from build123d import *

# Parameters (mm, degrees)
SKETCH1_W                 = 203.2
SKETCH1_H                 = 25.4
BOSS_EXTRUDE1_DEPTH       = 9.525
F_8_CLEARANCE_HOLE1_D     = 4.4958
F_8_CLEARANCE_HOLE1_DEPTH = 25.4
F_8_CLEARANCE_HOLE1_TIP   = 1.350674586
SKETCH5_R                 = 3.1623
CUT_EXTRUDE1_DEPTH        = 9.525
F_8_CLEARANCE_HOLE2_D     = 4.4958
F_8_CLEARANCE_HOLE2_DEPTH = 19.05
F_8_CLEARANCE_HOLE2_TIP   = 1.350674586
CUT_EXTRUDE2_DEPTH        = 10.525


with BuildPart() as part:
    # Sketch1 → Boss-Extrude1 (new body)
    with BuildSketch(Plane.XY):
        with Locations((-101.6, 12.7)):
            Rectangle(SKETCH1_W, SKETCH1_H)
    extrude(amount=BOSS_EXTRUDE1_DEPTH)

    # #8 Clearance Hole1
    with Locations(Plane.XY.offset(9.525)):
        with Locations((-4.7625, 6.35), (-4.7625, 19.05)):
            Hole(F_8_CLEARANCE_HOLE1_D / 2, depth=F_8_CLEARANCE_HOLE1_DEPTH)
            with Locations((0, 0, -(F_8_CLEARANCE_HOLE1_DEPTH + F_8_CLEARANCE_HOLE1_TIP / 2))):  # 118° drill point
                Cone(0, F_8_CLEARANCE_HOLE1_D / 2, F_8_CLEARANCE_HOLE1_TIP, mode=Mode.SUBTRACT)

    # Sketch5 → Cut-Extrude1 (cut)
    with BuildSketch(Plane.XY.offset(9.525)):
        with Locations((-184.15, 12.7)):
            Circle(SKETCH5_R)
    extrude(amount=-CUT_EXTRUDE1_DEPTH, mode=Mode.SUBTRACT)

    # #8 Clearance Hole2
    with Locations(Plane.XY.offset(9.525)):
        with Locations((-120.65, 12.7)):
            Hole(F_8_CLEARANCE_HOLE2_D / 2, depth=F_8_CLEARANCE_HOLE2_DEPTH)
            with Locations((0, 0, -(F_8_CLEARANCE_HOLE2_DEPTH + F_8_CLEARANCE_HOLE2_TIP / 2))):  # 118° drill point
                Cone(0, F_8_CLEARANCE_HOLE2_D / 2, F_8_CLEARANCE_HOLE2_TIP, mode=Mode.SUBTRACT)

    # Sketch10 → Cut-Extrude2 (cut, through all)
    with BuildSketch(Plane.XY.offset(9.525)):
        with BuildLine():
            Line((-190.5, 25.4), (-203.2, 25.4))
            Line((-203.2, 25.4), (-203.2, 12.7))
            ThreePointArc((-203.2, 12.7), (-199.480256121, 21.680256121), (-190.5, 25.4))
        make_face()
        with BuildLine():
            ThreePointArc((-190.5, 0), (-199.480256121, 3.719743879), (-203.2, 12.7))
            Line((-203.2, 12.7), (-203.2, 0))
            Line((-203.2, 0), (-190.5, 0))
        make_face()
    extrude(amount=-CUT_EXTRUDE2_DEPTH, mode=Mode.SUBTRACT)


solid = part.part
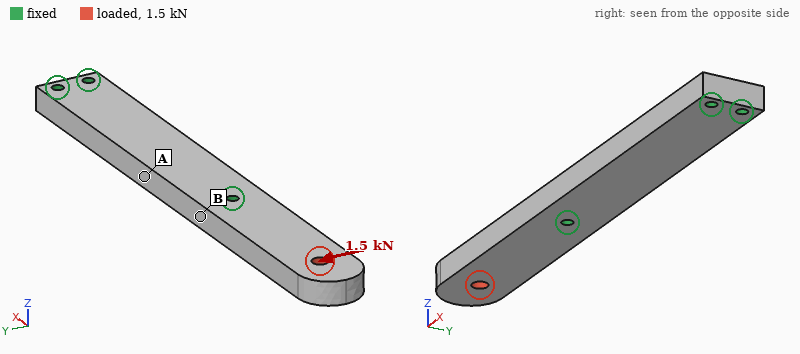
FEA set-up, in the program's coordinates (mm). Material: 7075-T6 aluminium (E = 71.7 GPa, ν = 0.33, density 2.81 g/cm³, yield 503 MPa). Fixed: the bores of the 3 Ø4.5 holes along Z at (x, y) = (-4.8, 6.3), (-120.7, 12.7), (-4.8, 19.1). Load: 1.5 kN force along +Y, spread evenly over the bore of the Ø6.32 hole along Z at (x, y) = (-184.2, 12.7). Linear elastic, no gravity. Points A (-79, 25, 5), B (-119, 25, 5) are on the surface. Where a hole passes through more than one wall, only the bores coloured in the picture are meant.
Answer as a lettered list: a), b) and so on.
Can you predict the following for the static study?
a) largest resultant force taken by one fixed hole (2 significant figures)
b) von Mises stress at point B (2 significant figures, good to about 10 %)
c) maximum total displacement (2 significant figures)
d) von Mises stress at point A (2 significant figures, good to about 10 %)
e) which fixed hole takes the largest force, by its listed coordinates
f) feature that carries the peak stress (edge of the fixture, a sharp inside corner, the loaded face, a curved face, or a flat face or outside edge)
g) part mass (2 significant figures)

a) 2.2 kN
b) 73 MPa
c) 0.39 mm
d) 28 MPa
e) (-120.7, 12.7)
f) edge of the fixture
g) 130 g
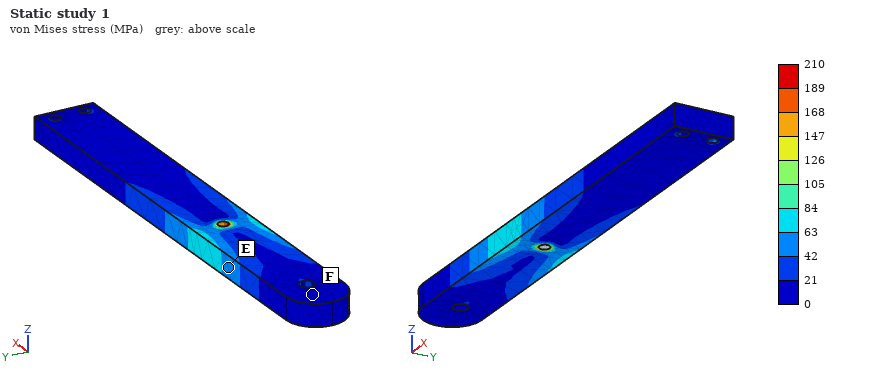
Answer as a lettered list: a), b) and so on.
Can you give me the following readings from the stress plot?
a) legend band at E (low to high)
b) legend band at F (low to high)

a) 42 to 63 MPa
b) 0 to 21 MPa
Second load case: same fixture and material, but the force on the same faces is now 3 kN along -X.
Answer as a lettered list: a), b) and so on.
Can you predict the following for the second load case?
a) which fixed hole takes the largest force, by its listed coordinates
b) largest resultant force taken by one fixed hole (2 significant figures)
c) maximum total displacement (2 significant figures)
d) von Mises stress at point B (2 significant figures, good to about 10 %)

a) (-120.7, 12.7)
b) 2.8 kN
c) 14 µm
d) 6.7 MPa
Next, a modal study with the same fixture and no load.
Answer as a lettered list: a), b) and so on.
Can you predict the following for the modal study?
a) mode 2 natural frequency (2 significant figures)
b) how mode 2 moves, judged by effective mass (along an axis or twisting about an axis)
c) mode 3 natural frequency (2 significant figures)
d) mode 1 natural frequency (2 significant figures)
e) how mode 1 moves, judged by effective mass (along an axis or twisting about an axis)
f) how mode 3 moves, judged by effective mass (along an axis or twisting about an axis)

a) 2200 Hz
b) along Y
c) 3500 Hz
d) 1200 Hz
e) along Z
f) along Z
